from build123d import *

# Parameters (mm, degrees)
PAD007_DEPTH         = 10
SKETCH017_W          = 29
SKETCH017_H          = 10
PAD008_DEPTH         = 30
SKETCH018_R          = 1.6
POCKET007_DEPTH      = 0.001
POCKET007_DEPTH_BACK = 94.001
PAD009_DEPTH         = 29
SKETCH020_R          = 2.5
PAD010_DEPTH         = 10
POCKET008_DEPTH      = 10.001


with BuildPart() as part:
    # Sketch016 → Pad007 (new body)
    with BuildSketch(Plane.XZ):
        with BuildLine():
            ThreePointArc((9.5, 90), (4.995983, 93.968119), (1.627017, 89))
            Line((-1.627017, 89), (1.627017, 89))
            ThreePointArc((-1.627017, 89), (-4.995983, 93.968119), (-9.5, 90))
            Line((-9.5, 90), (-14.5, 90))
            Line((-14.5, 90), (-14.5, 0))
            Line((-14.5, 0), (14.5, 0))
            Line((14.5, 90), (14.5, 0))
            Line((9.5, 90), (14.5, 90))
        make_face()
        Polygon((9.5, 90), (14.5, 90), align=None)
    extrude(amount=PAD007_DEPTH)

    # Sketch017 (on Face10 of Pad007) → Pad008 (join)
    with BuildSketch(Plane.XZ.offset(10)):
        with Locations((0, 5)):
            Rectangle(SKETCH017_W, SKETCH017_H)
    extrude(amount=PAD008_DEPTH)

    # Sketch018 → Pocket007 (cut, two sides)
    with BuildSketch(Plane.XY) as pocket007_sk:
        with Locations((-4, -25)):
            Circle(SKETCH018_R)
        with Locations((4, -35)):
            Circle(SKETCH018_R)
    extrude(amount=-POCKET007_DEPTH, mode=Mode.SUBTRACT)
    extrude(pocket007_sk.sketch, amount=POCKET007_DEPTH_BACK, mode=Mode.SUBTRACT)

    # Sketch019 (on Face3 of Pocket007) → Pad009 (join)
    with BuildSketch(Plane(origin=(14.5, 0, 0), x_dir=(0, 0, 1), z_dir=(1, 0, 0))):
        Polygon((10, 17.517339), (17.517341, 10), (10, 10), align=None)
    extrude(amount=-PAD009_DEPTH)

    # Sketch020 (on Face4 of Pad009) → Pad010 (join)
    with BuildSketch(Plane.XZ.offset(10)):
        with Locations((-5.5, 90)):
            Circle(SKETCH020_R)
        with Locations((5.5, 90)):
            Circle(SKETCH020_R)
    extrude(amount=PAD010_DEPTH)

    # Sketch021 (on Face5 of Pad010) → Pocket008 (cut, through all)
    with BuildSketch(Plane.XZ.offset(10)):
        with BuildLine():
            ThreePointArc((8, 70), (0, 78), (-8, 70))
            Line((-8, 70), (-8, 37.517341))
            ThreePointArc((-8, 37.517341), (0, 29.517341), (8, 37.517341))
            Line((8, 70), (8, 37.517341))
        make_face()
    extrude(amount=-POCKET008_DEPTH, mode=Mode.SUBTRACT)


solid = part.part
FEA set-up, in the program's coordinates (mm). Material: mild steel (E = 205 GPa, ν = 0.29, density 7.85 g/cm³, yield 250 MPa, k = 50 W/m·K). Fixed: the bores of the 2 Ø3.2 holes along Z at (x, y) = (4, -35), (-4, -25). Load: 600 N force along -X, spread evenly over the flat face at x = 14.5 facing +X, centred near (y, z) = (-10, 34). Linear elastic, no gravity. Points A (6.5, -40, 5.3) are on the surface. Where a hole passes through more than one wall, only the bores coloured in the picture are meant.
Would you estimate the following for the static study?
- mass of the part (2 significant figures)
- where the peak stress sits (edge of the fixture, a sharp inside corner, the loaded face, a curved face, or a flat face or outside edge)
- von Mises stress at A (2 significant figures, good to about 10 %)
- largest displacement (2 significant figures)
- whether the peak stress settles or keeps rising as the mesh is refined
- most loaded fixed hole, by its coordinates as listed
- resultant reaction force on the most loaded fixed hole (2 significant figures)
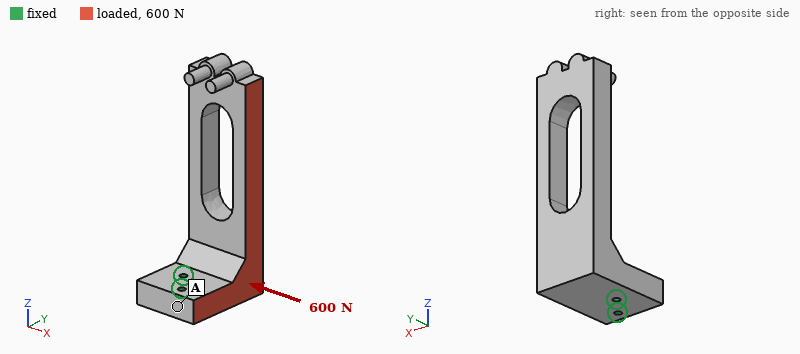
230 g
edge of the fixture
10 MPa
61 µm
keeps rising
(-4, -25)
1.1 kN
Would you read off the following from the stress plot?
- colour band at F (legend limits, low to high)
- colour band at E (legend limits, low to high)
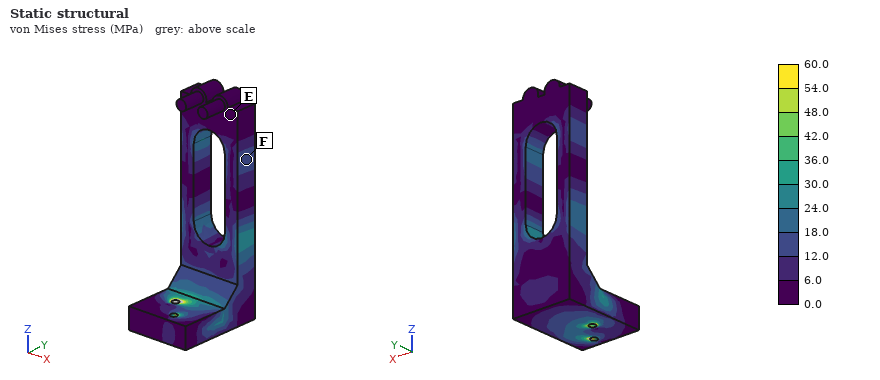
12.0 to 18.0 MPa
0.0 to 6.0 MPa
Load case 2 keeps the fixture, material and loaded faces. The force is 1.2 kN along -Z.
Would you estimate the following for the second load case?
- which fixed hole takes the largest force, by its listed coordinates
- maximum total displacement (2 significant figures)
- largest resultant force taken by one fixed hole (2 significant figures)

(-4, -25)
69 µm
910 N
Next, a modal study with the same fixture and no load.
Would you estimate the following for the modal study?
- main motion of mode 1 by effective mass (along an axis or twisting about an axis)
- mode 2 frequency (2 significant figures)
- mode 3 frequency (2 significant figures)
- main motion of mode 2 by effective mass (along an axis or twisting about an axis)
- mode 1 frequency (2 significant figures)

along Y
1300 Hz
3700 Hz
along X
900 Hz
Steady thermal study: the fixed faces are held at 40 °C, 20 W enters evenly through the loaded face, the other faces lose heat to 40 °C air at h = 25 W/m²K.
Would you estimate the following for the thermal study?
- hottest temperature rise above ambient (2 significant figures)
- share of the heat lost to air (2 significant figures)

53 K
28 %
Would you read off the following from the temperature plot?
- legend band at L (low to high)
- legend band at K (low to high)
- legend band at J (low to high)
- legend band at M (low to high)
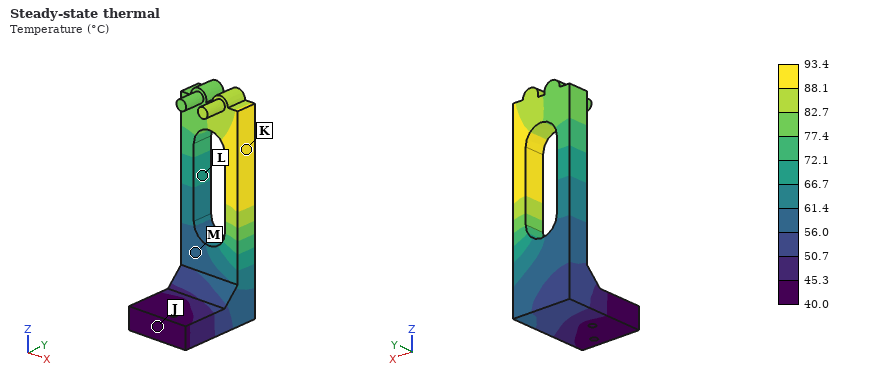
66.7 to 72.1 °C
88.1 to 93.4 °C
40.0 to 45.3 °C
56.0 to 61.4 °C
